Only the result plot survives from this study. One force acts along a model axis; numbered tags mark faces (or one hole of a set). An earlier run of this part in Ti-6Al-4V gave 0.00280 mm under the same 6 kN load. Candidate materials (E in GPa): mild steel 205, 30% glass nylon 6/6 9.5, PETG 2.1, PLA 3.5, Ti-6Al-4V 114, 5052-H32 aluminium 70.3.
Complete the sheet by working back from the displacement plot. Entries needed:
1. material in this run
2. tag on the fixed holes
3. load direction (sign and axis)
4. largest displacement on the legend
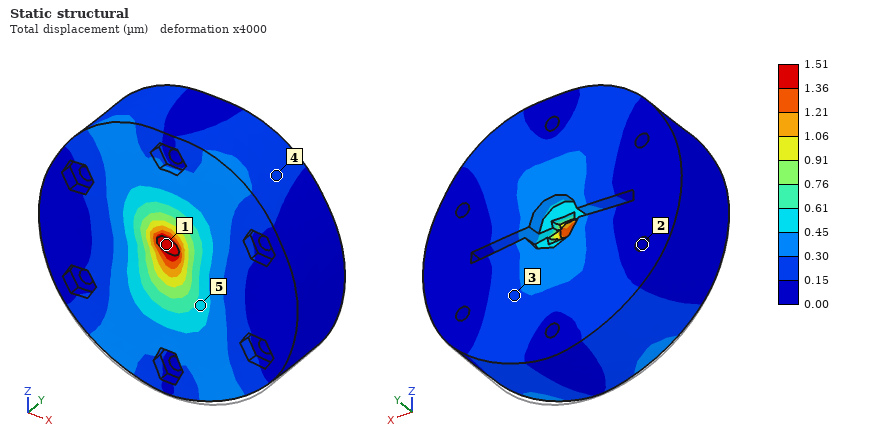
mild steel
2
+Z
1.51 µm
